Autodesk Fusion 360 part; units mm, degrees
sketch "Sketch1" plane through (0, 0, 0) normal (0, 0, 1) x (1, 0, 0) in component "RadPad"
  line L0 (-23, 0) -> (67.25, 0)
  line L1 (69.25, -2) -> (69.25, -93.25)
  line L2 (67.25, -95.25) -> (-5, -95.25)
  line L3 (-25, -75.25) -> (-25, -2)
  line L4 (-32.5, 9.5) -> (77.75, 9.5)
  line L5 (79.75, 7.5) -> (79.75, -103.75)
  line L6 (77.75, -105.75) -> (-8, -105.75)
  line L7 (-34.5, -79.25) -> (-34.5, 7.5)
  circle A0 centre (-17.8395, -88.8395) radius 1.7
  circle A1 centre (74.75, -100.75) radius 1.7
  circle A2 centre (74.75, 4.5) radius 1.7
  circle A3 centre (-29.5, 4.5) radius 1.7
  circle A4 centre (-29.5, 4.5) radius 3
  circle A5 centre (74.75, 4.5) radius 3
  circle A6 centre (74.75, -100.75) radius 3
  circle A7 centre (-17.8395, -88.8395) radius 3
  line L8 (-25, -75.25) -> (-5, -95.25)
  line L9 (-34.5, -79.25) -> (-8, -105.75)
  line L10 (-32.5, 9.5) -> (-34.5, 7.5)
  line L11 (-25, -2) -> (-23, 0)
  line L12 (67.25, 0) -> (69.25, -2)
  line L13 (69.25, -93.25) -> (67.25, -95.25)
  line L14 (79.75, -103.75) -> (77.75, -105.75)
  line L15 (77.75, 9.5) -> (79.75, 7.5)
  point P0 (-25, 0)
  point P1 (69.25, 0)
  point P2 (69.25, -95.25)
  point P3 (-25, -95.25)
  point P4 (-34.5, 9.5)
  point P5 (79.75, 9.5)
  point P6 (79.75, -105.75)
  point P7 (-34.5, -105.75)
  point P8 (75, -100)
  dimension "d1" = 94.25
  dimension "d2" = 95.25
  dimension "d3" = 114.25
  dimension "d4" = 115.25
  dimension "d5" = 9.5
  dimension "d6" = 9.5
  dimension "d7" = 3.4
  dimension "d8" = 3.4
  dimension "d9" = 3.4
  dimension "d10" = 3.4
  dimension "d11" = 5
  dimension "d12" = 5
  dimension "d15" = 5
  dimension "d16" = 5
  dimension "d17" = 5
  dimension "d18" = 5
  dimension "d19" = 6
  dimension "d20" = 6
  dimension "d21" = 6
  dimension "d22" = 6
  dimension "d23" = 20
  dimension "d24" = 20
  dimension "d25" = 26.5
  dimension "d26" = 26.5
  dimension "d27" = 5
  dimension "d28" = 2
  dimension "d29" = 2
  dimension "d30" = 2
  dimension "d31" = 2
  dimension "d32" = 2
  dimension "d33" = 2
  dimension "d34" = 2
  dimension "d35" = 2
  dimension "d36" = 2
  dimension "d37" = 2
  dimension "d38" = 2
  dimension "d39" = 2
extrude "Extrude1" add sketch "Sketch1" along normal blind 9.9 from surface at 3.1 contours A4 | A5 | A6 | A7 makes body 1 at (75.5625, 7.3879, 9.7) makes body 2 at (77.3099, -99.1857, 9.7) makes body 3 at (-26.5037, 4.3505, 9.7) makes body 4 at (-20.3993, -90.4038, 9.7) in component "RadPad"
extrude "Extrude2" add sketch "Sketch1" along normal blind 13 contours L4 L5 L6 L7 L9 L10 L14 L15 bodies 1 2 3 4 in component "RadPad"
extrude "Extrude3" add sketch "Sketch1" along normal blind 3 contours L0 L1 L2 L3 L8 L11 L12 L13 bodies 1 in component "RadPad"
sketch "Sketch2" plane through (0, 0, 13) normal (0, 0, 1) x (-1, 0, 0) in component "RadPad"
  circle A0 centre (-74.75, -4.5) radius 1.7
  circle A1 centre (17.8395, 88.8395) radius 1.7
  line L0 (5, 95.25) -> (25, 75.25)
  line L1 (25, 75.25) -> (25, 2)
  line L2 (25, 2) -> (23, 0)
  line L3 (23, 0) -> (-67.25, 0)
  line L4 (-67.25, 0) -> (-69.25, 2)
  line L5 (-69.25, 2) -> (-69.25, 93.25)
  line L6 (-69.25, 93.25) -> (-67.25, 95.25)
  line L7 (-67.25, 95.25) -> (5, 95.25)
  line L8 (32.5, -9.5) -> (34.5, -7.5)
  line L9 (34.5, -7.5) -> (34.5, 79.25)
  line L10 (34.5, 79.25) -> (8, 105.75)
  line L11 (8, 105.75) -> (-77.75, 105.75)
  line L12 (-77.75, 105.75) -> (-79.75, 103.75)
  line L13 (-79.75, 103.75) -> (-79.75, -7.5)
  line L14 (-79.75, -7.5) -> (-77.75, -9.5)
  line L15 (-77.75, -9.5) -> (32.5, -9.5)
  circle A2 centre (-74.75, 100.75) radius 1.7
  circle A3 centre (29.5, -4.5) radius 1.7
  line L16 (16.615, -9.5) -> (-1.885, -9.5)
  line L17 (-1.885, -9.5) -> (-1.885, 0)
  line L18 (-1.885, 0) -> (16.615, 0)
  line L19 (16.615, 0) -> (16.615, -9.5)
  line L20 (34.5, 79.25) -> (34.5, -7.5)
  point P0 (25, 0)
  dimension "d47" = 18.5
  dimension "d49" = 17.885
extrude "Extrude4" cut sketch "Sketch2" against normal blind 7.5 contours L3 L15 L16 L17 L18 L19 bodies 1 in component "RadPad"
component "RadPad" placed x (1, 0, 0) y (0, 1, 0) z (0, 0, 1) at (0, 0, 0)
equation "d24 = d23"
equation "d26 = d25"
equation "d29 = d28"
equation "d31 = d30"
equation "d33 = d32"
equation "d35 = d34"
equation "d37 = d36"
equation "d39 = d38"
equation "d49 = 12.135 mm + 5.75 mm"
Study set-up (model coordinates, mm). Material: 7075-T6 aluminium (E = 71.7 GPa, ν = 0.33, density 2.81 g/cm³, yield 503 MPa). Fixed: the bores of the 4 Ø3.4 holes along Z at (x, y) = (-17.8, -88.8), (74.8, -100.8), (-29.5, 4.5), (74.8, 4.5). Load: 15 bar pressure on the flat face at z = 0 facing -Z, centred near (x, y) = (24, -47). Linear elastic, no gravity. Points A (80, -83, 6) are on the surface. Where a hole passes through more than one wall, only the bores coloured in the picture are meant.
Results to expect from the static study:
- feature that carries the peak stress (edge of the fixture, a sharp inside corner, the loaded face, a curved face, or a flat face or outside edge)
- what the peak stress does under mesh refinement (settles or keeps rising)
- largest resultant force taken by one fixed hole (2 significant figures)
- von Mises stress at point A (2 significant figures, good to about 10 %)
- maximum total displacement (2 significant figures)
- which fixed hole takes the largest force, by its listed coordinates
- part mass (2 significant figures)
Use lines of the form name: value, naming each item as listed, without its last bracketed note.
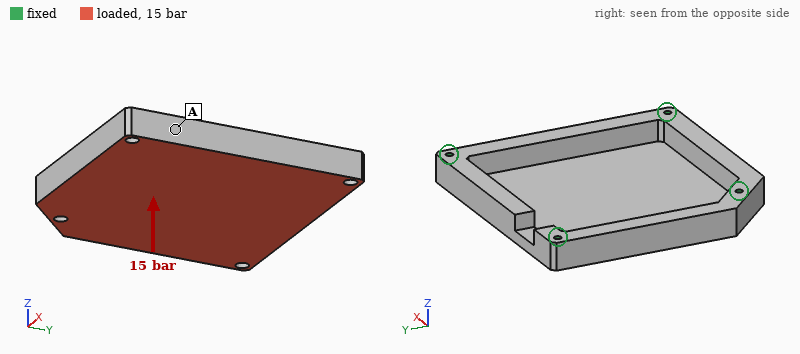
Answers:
feature that carries the peak stress: edge of the fixture
what the peak stress does under mesh refinement: keeps rising
largest resultant force taken by one fixed hole: 7.5 kN
von Mises stress at point A: 52 MPa
maximum total displacement: 1.4 mm
which fixed hole takes the largest force, by its listed coordinates: (74.8, 4.5)
part mass: 220 g
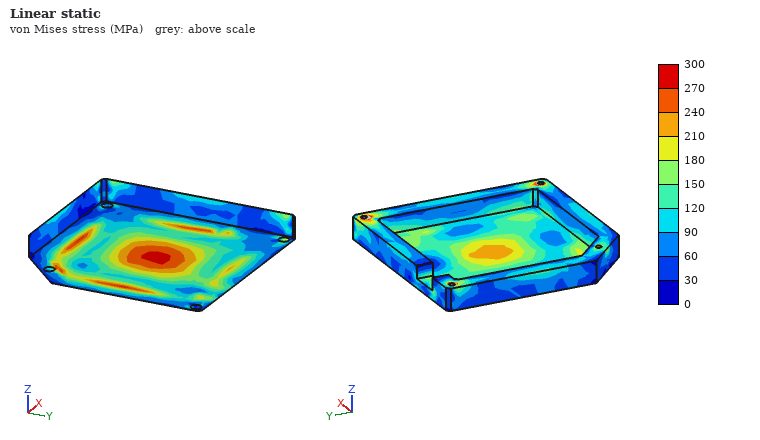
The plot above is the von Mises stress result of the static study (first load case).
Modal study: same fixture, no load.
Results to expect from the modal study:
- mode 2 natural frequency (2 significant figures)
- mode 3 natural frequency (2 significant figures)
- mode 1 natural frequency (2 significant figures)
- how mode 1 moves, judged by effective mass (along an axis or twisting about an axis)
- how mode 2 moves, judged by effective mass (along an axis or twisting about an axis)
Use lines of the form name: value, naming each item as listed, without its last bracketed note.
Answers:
mode 2 natural frequency: 3900 Hz
mode 3 natural frequency: 4300 Hz
mode 1 natural frequency: 2300 Hz
how mode 1 moves, judged by effective mass: along Z
how mode 2 moves, judged by effective mass: twisting about X
